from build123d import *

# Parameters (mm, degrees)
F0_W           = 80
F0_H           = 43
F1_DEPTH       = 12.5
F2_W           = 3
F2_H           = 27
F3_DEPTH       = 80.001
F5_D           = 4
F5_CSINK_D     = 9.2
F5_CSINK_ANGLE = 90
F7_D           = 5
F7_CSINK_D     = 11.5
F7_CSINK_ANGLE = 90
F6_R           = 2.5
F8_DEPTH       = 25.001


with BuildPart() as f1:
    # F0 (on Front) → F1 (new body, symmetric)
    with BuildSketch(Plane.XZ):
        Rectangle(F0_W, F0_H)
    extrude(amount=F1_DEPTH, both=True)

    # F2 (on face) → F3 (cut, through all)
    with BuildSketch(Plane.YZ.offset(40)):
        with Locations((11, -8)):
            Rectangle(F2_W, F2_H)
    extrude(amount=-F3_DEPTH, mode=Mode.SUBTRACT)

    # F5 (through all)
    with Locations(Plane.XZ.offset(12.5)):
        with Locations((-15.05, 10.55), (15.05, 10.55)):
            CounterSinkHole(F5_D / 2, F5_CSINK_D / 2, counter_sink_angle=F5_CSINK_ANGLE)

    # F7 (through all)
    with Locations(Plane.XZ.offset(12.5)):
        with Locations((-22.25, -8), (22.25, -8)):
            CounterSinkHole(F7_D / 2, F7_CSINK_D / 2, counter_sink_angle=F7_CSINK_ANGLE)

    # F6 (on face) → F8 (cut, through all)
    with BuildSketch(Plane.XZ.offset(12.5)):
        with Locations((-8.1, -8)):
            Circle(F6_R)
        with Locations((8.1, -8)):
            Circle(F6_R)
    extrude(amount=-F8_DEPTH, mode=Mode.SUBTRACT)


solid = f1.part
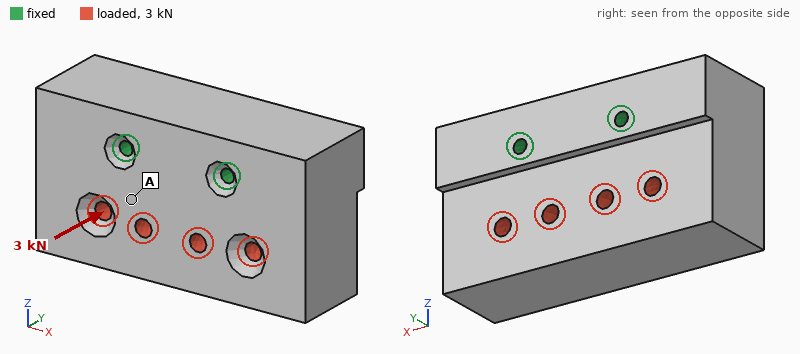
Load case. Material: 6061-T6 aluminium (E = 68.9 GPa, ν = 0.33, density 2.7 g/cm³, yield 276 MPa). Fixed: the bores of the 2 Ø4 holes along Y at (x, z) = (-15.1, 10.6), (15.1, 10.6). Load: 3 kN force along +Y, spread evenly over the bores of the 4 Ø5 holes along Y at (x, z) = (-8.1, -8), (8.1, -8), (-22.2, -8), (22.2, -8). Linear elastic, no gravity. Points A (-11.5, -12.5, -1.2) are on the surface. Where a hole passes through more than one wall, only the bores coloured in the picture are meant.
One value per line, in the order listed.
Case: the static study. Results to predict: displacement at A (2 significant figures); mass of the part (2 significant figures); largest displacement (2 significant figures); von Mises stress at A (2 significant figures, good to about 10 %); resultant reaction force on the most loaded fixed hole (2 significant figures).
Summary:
4.5 µm
210 g
9.5 µm
4.2 MPa
1.5 kN
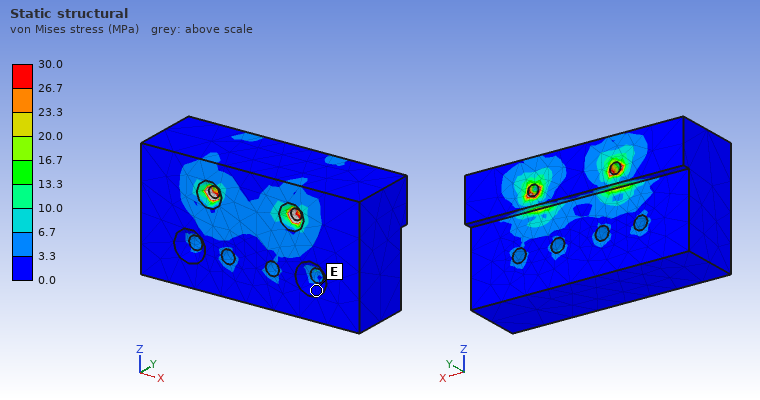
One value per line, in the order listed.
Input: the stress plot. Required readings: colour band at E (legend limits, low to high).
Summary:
0.0 to 3.3 MPa
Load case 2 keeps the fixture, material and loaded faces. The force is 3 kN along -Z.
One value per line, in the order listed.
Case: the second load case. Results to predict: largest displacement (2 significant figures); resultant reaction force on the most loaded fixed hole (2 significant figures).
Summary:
1.2 µm
1.5 kN
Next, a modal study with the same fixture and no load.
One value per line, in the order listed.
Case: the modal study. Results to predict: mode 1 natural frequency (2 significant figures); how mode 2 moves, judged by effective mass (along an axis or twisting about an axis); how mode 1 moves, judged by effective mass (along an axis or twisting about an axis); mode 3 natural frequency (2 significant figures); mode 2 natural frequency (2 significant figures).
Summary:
9200 Hz
along X
along Y
11 kHz
10 kHz
